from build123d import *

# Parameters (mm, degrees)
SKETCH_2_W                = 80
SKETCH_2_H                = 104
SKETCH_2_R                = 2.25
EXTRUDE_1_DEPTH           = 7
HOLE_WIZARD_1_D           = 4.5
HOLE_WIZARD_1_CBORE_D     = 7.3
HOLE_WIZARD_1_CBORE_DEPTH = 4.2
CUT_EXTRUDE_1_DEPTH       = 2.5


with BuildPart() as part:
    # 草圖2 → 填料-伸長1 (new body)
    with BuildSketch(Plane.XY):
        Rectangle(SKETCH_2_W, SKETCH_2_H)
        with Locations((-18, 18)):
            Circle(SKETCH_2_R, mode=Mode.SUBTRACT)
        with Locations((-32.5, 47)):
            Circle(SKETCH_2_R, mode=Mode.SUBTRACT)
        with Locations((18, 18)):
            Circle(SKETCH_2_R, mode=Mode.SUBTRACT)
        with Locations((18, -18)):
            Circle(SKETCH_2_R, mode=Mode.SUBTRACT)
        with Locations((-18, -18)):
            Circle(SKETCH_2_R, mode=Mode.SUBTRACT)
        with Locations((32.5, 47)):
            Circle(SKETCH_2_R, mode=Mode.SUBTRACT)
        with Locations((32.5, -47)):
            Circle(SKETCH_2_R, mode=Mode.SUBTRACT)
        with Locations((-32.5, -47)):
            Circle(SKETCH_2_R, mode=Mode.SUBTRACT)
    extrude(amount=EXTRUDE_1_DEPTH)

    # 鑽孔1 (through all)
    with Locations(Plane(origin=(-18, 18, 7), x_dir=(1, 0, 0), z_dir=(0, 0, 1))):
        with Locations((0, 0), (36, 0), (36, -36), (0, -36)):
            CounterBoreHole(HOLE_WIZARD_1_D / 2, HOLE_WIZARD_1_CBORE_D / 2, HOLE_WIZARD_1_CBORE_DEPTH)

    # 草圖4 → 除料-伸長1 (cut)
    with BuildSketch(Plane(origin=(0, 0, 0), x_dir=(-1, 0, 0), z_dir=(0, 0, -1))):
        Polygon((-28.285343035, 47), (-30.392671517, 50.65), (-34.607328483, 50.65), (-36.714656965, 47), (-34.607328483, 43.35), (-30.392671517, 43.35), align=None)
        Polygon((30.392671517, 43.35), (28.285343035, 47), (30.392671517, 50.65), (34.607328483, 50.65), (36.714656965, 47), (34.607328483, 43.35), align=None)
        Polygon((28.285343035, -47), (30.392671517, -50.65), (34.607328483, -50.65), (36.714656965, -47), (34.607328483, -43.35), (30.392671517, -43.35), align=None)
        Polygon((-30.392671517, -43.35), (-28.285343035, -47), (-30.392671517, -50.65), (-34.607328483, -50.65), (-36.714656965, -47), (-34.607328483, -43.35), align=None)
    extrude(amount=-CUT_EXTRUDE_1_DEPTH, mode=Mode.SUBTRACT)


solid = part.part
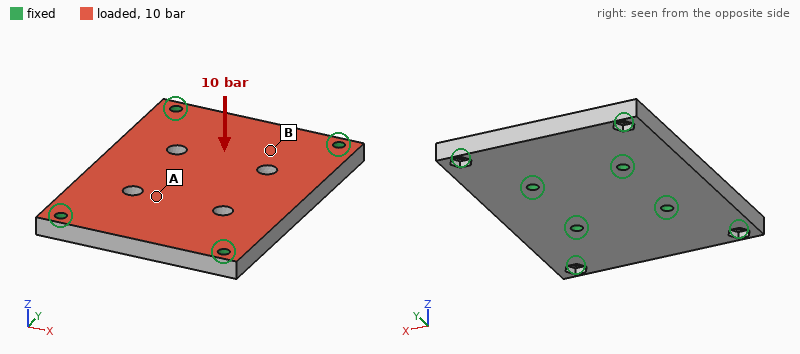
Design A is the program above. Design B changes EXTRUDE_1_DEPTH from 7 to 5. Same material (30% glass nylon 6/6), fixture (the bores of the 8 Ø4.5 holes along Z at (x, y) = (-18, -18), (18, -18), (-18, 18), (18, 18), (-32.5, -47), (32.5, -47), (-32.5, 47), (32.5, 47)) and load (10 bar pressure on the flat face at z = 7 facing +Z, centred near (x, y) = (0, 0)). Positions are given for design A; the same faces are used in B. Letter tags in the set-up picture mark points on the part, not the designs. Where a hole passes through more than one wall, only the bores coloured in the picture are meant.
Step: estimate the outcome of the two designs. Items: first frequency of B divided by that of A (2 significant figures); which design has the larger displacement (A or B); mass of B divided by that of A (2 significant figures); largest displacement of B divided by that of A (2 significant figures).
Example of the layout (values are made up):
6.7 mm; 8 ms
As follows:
0.77; B; 0.71; 2.6
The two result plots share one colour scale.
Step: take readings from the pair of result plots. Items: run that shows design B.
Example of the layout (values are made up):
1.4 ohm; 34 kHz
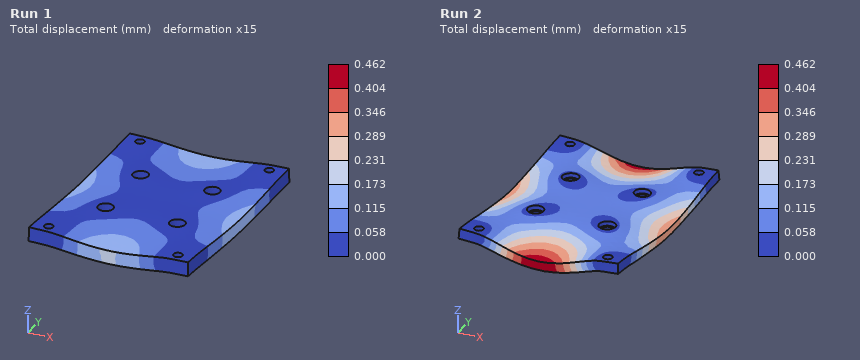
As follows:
Run 2
